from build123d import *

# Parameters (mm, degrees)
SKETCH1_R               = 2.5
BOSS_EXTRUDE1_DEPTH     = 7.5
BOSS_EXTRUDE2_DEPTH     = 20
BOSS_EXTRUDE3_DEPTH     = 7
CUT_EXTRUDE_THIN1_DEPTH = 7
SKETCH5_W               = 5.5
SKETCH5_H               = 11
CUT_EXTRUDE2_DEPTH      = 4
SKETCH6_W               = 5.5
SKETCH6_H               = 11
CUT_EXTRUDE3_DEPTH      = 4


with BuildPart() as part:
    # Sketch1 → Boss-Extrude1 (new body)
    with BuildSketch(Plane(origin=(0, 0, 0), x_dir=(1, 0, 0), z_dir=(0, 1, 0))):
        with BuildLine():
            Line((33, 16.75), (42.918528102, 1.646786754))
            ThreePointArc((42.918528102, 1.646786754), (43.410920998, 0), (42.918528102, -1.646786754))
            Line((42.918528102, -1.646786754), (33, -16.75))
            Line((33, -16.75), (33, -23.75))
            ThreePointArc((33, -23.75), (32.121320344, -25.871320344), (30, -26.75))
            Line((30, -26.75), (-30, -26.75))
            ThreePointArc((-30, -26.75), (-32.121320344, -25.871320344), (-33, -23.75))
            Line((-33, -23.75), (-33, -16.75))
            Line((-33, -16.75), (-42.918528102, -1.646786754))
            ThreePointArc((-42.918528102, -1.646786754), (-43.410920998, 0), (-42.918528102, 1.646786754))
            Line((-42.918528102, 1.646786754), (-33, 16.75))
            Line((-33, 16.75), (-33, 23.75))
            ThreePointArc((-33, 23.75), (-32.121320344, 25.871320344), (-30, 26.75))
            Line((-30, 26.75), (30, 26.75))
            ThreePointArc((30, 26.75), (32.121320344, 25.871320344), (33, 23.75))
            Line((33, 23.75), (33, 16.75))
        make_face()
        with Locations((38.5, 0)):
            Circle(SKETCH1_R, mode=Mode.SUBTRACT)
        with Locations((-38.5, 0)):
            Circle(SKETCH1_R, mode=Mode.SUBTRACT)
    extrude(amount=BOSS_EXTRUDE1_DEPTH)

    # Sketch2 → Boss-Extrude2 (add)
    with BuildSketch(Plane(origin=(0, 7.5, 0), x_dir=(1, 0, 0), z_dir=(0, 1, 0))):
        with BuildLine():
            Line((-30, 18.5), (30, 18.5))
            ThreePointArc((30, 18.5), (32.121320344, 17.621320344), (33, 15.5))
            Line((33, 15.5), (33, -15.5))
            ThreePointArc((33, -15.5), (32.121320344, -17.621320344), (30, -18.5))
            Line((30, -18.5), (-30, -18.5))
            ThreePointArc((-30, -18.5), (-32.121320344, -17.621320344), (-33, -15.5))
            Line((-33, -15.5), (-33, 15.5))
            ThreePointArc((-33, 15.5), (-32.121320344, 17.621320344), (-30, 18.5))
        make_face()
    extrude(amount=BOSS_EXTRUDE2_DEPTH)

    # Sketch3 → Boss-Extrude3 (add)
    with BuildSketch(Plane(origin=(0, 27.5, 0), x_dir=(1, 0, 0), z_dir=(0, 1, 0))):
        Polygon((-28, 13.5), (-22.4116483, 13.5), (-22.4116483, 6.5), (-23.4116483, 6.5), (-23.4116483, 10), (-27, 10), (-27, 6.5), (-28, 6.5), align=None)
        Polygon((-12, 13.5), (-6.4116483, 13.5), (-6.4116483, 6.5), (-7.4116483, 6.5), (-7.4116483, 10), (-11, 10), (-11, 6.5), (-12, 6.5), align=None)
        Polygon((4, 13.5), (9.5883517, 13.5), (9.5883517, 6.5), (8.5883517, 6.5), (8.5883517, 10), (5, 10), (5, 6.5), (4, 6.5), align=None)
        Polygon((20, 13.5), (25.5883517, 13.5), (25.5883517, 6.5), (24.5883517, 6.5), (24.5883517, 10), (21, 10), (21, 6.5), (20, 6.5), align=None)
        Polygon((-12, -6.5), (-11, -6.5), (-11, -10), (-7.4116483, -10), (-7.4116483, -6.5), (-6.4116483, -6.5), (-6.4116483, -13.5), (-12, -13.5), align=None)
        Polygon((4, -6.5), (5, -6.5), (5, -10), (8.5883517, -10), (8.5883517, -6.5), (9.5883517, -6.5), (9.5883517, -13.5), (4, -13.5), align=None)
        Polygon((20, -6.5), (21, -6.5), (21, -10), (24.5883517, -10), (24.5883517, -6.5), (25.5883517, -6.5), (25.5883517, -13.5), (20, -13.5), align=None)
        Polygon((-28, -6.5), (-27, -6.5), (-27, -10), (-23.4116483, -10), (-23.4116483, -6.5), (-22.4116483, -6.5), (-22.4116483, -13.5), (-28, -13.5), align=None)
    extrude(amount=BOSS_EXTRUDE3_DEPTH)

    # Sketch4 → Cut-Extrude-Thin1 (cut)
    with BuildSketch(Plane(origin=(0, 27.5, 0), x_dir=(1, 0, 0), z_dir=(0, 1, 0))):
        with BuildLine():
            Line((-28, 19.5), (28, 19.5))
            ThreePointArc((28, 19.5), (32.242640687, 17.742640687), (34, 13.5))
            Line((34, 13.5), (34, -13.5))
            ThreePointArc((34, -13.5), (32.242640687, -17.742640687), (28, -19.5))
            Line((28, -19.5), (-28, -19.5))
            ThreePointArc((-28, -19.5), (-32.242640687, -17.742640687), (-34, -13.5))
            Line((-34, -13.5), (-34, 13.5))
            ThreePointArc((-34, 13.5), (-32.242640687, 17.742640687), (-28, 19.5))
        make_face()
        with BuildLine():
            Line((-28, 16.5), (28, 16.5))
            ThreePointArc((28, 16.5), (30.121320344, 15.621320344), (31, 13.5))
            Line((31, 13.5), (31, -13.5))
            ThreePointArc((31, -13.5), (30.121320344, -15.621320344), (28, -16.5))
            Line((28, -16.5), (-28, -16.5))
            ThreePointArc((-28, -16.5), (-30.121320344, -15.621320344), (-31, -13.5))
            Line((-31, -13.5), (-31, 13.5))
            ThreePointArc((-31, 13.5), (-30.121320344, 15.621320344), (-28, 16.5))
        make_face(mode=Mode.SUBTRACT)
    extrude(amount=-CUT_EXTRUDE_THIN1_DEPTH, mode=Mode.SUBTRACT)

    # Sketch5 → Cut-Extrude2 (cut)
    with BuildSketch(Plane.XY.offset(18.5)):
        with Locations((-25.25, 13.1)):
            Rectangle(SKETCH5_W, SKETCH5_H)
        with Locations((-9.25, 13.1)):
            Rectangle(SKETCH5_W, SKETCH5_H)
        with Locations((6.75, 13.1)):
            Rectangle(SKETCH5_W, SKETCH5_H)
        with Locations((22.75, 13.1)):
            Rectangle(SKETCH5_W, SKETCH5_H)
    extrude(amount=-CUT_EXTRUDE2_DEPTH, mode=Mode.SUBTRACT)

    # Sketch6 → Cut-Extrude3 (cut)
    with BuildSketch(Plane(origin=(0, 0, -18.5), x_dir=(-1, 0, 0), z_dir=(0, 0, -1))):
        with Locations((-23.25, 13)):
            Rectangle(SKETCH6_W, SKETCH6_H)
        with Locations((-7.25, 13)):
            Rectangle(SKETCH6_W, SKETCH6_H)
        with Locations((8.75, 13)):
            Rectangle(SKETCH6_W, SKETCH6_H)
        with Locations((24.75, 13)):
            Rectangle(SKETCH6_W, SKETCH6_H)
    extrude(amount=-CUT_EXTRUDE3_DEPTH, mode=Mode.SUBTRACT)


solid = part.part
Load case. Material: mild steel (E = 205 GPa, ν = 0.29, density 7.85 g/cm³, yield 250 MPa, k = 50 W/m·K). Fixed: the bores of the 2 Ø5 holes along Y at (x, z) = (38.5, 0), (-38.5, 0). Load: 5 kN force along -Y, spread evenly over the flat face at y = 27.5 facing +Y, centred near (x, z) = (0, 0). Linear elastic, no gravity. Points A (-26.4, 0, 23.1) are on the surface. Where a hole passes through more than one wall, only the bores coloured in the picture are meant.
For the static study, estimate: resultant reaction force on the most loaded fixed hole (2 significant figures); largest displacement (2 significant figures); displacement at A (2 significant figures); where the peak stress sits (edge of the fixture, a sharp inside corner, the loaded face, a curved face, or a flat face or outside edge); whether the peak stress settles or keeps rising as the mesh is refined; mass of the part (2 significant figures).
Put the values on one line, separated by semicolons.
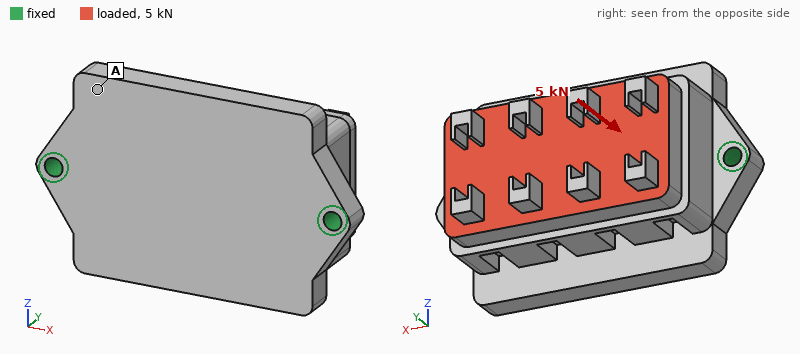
2.8 kN; 5.3 µm; 4.2 µm; edge of the fixture; keeps rising; 580 g
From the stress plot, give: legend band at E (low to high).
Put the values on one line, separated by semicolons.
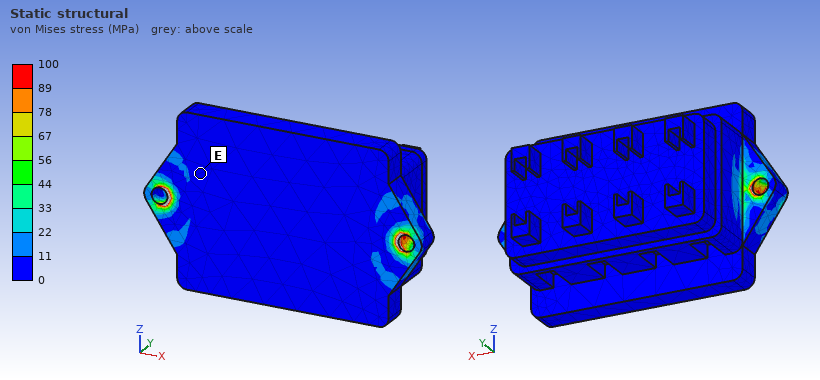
0 to 11 MPa
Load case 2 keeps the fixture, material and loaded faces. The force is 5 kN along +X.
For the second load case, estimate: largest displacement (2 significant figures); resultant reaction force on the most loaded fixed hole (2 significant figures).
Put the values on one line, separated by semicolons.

4.0 µm; 3.0 kN
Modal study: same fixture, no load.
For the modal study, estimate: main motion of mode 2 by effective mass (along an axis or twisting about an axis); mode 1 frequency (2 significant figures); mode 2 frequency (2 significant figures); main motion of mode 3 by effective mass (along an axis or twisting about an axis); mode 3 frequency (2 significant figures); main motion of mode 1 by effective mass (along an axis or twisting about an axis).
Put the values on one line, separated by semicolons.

along Y; 2700 Hz; 7000 Hz; along Z; 10 kHz; along Z
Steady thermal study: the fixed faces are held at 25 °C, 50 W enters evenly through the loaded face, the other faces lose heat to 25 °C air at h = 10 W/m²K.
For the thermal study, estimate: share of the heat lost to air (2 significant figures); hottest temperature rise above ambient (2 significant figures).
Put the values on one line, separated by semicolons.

9.7 %; 44 K
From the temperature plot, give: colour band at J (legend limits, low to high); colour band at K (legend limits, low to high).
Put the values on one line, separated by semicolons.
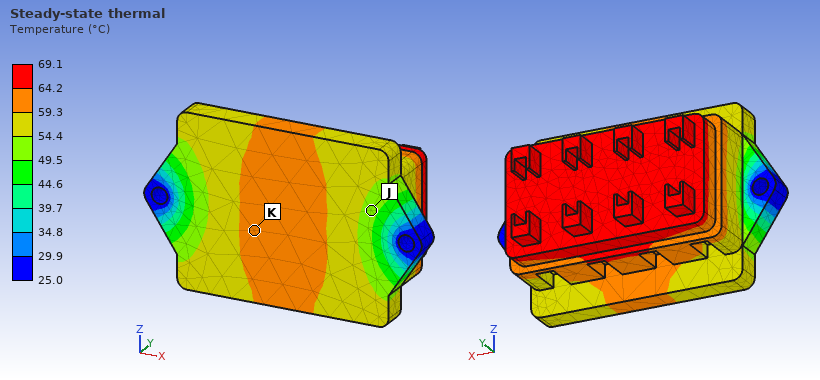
49.5 to 54.4 °C; 59.3 to 64.2 °C
